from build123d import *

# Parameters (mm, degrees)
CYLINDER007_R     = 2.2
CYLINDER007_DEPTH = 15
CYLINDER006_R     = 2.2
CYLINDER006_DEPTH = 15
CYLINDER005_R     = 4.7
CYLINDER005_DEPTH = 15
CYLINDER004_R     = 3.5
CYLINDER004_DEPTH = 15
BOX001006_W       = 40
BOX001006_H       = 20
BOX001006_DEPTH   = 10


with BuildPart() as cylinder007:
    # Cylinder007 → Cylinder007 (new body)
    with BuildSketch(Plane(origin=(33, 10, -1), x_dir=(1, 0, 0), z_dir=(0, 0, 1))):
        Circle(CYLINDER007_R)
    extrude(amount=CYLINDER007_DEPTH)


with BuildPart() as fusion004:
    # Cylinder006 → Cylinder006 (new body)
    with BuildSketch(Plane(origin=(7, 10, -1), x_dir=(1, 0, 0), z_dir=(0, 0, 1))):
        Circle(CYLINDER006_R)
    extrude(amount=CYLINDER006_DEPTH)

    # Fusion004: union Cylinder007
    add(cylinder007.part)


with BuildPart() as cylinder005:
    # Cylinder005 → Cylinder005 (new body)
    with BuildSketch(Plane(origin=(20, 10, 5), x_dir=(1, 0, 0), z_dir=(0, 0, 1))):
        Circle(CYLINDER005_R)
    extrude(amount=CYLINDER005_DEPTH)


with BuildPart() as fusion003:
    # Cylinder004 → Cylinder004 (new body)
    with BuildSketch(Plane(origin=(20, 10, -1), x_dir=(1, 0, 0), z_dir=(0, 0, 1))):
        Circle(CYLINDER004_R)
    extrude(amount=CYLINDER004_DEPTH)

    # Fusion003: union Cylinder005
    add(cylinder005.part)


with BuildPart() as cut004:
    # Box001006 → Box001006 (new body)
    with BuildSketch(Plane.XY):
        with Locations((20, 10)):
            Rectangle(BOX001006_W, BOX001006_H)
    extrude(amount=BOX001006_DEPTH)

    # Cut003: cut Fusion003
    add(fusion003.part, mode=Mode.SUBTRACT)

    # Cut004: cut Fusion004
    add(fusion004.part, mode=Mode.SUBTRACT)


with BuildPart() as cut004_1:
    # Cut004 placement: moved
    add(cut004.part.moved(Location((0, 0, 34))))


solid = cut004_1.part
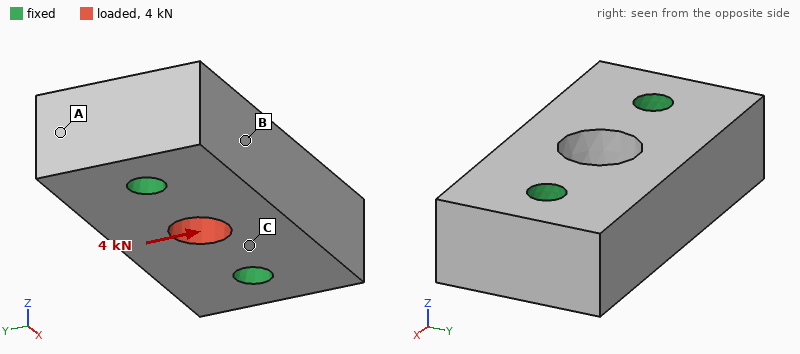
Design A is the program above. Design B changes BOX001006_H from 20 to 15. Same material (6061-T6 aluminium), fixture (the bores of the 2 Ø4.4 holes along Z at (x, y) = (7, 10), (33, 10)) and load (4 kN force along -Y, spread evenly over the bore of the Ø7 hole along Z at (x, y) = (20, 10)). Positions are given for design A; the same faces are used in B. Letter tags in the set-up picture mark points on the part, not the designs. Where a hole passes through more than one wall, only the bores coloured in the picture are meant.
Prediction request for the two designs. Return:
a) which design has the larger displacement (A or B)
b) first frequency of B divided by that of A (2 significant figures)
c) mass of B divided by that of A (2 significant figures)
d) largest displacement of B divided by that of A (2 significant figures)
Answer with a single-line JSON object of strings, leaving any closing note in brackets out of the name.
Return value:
{"which design has the larger displacement": "B", "first frequency of B divided by that of A": "1.3", "mass of B divided by that of A": "0.72", "largest displacement of B divided by that of A": "1.4"}
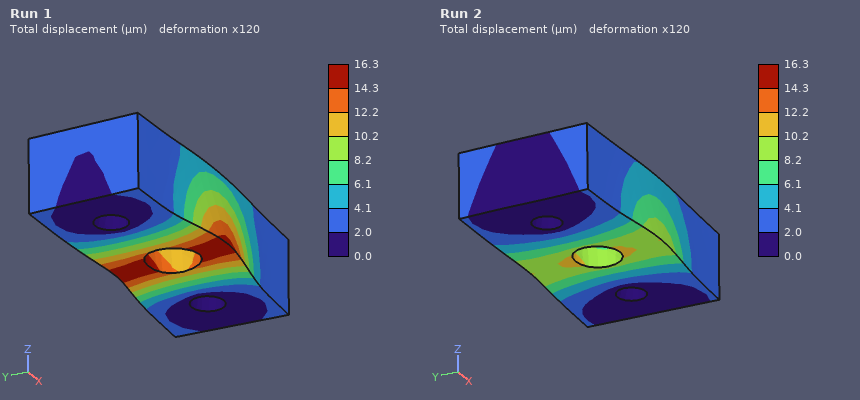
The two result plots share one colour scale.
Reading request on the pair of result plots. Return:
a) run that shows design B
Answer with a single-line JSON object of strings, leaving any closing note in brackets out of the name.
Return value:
{"run that shows design B": "Run 1"}
